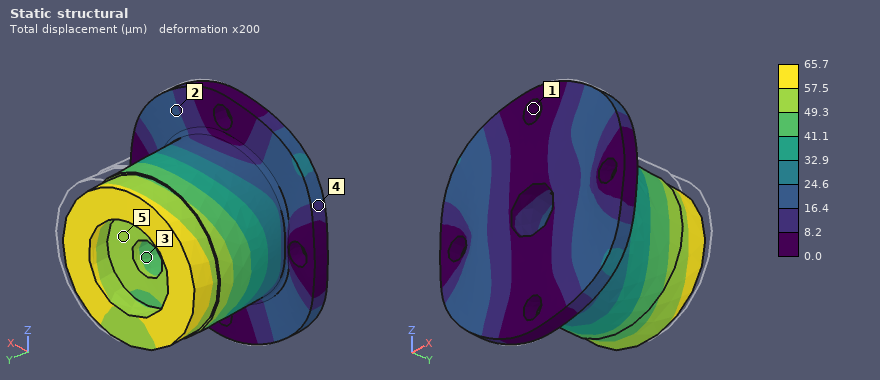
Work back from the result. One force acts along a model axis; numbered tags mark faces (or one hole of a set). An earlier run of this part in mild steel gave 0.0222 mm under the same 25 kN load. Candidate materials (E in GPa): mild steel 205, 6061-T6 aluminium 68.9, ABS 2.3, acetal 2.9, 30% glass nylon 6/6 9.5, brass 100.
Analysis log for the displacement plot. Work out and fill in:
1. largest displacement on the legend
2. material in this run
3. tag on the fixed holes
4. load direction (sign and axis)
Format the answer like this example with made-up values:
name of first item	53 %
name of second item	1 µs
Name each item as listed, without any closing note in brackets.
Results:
largest displacement on the legend	65.7 µm
material in this run	6061-T6 aluminium
tag on the fixed holes	1
load direction	-X
